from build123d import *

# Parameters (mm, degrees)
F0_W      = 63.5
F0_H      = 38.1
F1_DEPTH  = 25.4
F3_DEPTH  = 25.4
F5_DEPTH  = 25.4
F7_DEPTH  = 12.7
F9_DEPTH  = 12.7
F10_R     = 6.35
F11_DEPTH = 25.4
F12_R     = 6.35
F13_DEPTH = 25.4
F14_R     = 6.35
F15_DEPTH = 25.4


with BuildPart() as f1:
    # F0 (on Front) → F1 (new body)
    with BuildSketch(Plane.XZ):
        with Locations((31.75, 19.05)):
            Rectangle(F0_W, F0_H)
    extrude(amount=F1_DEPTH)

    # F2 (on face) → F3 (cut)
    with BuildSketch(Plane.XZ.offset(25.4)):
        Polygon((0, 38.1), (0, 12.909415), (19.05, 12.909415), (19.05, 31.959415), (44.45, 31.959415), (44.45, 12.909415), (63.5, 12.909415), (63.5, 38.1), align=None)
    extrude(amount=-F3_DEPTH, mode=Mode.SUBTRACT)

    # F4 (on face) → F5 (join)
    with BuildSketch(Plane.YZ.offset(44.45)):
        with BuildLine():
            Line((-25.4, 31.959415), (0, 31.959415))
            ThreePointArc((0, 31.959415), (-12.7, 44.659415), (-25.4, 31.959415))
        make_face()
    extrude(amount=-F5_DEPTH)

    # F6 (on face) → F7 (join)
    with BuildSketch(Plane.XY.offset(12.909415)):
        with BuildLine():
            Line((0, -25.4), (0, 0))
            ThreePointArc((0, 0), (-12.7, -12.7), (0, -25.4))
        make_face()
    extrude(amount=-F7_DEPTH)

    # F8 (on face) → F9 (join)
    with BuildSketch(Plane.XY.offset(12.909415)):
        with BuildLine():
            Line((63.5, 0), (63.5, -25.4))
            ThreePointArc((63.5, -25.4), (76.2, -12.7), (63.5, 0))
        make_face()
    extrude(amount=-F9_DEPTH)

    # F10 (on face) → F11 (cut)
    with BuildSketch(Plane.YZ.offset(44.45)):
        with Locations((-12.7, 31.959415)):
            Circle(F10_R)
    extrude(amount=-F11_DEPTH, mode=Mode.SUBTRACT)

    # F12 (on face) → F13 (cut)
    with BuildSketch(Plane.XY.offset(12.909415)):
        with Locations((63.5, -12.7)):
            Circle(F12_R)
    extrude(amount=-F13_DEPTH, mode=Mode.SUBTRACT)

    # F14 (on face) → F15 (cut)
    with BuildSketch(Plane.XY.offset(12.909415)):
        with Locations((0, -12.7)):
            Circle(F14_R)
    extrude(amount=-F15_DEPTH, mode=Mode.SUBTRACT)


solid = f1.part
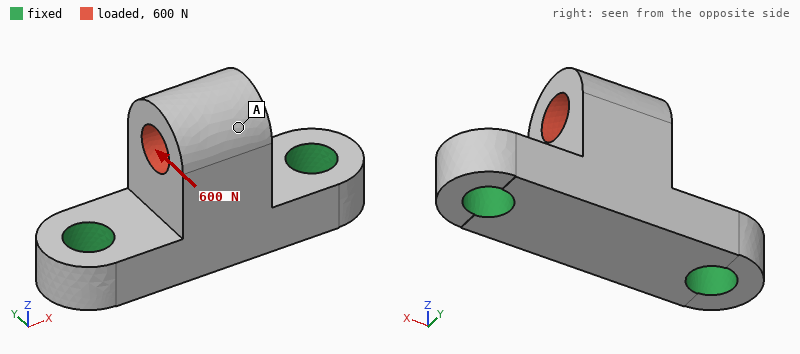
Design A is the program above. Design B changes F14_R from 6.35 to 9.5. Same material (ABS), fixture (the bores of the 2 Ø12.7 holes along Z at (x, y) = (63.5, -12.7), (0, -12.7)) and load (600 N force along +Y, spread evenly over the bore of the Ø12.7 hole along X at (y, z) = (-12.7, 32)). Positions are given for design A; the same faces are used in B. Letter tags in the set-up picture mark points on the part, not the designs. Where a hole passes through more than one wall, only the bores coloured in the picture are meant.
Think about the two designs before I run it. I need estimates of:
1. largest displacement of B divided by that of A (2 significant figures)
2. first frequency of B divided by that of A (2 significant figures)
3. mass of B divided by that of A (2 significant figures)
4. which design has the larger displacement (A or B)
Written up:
0.88
1.1
0.95
A
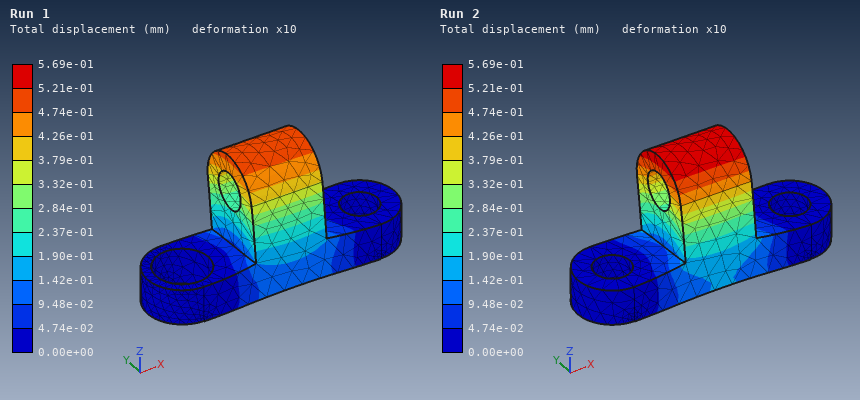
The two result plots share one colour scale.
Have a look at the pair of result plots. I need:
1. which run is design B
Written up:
Run 1
